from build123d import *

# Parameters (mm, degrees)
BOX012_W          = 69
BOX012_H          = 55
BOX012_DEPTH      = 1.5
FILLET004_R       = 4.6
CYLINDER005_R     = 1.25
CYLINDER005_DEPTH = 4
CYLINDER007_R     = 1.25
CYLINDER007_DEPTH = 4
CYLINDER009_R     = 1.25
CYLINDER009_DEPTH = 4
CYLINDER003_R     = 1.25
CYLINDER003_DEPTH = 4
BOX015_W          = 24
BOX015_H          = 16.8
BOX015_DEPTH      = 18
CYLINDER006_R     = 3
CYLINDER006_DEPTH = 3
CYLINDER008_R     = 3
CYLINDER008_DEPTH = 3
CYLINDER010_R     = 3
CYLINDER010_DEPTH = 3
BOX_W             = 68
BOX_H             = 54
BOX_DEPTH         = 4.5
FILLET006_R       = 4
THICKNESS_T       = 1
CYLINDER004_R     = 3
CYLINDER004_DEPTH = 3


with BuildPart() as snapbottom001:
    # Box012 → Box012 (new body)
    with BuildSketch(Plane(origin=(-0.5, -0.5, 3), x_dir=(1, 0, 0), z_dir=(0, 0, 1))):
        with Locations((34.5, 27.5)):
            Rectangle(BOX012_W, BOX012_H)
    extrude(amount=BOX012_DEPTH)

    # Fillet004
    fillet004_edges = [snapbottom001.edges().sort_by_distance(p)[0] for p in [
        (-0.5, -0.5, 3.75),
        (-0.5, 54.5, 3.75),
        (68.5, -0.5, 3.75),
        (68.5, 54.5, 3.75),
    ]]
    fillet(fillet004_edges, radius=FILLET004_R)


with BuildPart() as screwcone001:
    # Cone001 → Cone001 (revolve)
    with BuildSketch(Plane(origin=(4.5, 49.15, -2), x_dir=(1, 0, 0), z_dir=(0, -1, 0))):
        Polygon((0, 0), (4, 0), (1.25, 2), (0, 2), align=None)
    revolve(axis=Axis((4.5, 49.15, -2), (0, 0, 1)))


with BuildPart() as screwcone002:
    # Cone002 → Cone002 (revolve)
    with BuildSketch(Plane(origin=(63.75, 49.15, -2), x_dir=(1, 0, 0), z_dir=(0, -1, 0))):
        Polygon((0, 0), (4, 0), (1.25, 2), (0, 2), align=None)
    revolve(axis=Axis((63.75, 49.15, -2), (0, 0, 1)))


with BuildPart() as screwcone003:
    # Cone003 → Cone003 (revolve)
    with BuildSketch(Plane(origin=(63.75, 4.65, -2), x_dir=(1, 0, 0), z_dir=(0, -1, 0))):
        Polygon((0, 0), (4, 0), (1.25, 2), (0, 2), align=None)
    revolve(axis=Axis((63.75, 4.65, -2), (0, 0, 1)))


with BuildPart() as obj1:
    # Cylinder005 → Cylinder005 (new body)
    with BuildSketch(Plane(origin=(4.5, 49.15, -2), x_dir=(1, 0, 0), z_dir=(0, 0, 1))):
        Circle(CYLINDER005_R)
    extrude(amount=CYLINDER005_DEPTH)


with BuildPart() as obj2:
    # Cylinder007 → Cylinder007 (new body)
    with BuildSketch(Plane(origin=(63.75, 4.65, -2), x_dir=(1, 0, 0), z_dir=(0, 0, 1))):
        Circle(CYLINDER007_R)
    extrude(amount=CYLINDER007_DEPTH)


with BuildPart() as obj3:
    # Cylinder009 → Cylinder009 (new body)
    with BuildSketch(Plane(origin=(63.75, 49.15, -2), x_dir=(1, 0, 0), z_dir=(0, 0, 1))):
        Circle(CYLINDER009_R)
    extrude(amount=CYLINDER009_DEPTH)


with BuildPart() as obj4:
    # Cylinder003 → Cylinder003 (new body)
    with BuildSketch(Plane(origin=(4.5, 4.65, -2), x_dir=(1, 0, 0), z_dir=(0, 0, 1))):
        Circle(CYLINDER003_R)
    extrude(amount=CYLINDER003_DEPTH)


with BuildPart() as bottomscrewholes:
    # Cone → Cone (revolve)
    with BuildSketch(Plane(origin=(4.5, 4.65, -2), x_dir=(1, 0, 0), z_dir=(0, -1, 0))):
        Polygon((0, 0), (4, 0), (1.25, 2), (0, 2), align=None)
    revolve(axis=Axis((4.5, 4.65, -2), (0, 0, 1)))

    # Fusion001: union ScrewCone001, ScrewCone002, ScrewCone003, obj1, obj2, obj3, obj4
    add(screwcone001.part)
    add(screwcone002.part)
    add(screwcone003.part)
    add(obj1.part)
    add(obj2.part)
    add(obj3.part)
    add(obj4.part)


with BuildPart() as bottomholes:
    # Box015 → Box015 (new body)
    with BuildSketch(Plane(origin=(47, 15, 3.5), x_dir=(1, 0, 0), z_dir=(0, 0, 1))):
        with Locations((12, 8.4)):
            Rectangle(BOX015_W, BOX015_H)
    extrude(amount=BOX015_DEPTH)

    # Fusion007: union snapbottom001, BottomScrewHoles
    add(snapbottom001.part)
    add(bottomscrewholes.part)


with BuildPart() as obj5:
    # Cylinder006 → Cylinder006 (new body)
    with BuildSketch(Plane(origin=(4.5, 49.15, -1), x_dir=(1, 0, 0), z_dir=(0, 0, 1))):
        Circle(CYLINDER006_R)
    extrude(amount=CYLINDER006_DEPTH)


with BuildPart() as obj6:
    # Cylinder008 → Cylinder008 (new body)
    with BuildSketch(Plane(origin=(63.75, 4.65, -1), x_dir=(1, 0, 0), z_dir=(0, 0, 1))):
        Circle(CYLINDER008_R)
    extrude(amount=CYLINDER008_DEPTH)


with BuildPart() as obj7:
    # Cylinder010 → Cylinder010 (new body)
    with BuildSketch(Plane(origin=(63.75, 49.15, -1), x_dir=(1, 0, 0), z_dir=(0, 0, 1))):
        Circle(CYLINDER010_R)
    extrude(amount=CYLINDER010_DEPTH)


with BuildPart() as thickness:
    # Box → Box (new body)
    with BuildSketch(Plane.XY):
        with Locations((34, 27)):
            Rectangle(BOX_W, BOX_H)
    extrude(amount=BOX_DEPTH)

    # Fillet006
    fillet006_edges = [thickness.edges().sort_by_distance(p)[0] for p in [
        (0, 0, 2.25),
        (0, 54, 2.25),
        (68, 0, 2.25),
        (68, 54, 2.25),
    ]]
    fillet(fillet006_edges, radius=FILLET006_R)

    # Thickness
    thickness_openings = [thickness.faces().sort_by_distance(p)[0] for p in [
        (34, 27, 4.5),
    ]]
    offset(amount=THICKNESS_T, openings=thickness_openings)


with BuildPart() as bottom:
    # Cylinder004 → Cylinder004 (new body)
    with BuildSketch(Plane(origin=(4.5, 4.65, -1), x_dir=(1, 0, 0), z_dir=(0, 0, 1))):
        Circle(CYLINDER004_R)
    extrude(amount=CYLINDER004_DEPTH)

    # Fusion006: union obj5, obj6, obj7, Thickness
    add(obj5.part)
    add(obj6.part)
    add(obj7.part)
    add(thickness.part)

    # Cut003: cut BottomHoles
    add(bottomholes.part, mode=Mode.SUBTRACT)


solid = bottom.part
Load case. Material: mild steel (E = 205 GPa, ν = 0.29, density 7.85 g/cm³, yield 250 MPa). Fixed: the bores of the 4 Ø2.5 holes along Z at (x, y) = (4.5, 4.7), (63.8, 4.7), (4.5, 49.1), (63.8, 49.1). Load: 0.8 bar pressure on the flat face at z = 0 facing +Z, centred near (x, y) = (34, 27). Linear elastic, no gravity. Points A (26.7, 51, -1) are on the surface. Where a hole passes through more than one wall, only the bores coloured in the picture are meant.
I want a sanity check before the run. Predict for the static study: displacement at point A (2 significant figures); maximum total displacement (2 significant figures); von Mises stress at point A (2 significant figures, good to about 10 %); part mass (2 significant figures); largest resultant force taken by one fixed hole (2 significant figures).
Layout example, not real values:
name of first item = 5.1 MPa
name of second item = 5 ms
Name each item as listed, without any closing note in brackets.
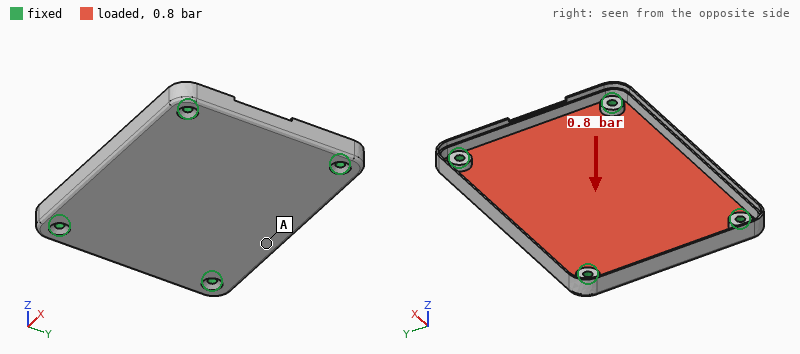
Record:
displacement at point A = 0.039 mm
maximum total displacement = 0.14 mm
von Mises stress at point A = 28 MPa
part mass = 38 g
largest resultant force taken by one fixed hole = 90 N
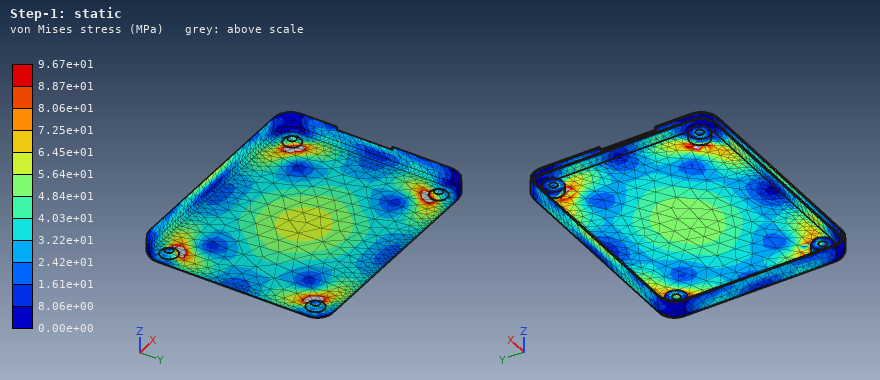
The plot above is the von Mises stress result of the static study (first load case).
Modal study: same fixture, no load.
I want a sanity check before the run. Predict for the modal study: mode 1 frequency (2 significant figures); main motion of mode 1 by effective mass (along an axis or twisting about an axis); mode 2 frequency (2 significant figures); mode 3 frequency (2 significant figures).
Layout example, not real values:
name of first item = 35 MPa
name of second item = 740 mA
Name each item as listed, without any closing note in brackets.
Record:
mode 1 frequency = 1700 Hz
main motion of mode 1 by effective mass = along Z
mode 2 frequency = 3400 Hz
mode 3 frequency = 3500 Hz
